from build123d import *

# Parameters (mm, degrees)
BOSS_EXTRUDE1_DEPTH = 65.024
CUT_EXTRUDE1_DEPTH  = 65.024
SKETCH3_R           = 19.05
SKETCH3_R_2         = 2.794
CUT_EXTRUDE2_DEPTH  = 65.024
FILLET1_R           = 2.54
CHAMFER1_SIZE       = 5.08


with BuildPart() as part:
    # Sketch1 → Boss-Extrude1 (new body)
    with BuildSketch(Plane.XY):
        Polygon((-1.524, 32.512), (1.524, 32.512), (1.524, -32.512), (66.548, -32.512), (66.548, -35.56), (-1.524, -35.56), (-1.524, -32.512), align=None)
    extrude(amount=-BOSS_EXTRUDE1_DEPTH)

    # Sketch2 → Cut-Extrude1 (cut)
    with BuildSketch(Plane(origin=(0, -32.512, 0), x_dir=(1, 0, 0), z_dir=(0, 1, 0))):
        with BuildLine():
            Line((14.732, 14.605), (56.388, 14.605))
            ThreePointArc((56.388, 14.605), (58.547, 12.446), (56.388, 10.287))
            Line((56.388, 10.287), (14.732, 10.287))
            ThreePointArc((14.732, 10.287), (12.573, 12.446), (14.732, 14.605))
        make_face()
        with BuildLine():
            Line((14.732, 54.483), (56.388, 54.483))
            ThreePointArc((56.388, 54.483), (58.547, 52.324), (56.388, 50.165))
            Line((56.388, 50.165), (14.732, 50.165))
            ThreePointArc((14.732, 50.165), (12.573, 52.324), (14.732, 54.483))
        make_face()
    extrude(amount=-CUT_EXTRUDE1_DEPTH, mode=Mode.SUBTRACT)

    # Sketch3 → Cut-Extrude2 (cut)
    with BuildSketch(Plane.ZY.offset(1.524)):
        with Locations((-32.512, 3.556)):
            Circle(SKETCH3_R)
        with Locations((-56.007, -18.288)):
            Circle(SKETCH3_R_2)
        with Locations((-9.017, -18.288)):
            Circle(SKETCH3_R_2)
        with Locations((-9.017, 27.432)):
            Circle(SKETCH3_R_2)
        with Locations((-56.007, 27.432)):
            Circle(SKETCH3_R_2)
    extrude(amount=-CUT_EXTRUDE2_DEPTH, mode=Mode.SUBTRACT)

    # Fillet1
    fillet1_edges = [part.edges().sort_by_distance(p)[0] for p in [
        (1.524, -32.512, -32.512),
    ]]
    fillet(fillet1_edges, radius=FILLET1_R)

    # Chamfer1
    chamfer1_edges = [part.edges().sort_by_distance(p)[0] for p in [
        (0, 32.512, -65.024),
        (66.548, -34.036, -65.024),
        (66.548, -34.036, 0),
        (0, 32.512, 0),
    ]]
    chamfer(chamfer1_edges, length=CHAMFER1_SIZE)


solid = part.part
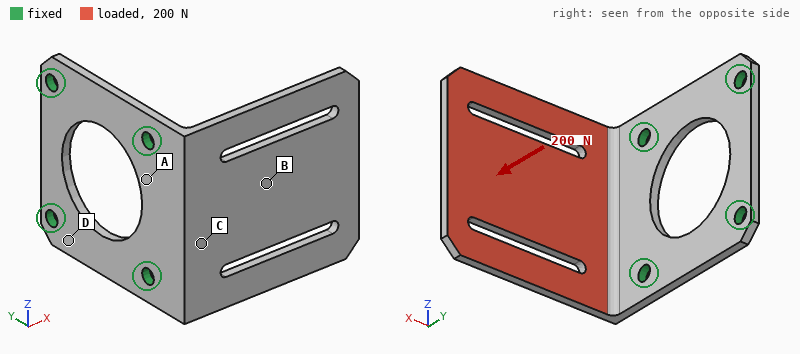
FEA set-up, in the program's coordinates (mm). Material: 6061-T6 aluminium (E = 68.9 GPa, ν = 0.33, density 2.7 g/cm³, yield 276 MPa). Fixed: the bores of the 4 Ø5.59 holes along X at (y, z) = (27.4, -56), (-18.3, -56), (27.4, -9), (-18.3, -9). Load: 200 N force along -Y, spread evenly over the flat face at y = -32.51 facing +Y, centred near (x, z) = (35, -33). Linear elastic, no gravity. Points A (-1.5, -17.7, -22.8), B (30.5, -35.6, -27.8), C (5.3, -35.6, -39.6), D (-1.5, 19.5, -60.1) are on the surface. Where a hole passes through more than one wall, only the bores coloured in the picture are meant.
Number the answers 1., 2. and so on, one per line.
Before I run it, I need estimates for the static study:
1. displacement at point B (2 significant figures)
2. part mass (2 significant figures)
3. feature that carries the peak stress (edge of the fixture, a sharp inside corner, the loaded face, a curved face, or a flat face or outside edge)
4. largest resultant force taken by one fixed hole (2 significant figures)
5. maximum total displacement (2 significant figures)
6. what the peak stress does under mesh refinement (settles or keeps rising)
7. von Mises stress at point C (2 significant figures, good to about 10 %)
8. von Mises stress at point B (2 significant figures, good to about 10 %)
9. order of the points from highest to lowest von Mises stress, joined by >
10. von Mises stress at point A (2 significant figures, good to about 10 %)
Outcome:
1. 0.49 mm
2. 58 g
3. edge of the fixture
4. 110 N
5. 1.3 mm
6. keeps rising
7. 55 MPa
8. 22 MPa
9. C > A > B > D
10. 37 MPa
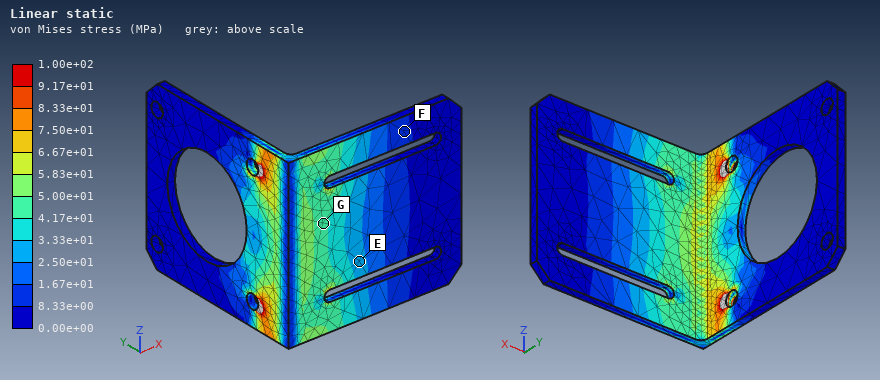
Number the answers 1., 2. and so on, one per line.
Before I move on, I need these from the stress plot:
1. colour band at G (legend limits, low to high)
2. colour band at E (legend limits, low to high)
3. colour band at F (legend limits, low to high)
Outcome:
1. 4.17e+01 to 5.00e+01 MPa
2. 2.50e+01 to 3.33e+01 MPa
3. 8.33e+00 to 1.67e+01 MPa
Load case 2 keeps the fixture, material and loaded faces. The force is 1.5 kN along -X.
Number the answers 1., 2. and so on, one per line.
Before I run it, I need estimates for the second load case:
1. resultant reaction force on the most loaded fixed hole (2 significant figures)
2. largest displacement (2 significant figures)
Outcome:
1. 760 N
2. 0.67 mm
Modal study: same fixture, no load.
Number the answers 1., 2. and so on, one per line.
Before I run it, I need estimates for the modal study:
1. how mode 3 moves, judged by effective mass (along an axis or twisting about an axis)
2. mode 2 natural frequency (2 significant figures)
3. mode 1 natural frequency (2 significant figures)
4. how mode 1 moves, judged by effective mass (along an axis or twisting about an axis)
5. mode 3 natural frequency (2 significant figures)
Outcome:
1. along Z
2. 1200 Hz
3. 440 Hz
4. along Y
5. 1900 Hz
